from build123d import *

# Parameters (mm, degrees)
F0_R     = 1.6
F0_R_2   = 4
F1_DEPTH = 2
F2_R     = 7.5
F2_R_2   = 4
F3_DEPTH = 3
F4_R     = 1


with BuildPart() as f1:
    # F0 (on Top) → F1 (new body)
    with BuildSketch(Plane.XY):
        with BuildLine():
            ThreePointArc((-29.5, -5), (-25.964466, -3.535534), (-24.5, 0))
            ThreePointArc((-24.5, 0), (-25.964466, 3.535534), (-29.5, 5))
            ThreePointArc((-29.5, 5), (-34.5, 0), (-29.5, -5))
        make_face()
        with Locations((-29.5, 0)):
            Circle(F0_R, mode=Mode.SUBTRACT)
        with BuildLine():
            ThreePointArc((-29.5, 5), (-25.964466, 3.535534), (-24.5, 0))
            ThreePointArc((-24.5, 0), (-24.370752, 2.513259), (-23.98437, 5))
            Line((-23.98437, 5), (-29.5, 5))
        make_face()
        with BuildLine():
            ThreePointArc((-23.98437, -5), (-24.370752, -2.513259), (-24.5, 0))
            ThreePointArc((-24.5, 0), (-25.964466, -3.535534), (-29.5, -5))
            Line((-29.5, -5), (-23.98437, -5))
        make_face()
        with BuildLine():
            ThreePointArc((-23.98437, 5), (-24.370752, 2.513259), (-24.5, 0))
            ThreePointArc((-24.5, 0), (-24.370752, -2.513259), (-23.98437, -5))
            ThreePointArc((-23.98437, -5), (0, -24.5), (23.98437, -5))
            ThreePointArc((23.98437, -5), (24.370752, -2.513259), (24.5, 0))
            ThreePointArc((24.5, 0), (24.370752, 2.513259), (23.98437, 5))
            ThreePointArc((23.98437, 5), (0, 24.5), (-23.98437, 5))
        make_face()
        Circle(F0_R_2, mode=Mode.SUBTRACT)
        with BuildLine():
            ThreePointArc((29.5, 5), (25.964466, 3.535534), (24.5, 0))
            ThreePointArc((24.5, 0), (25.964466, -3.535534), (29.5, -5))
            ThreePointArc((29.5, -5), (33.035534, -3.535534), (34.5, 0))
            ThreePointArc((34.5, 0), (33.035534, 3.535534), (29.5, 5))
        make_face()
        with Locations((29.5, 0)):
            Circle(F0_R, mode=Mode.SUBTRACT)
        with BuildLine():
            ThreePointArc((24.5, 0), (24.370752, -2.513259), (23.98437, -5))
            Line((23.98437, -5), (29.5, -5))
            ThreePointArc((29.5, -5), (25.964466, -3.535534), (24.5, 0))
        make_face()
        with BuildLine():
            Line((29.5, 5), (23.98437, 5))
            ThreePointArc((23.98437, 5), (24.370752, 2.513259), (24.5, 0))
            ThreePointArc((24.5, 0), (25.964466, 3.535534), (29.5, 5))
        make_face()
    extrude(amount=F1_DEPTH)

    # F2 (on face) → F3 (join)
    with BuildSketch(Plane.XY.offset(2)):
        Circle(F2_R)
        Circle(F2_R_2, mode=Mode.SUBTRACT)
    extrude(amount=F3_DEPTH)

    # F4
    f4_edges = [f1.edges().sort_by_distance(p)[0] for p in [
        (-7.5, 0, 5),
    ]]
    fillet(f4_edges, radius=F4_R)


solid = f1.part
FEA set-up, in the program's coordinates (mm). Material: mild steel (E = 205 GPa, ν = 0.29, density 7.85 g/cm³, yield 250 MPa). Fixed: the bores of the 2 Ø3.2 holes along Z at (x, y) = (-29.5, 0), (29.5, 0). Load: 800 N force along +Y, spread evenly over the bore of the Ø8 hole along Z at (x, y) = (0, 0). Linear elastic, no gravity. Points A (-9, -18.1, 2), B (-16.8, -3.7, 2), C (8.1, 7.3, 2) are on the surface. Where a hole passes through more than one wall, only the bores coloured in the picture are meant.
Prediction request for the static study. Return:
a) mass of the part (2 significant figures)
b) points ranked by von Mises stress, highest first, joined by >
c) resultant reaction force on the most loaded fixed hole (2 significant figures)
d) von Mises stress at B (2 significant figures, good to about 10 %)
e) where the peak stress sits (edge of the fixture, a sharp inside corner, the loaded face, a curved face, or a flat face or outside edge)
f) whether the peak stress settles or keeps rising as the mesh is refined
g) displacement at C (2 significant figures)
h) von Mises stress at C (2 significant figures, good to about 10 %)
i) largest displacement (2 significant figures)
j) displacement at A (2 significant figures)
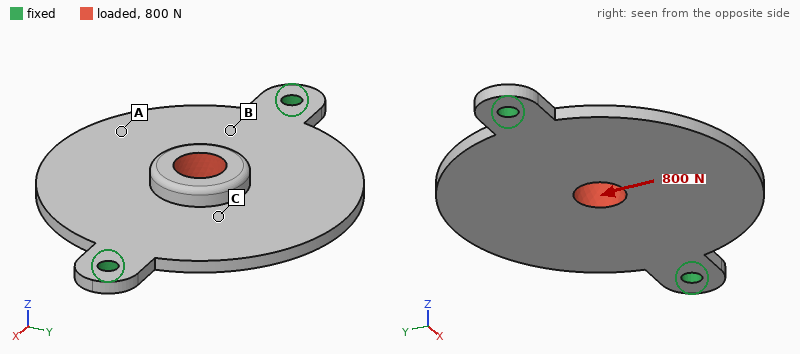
34 g
B > C > A
400 N
36 MPa
edge of the fixture
keeps rising
25 µm
21 MPa
81 µm
58 µm
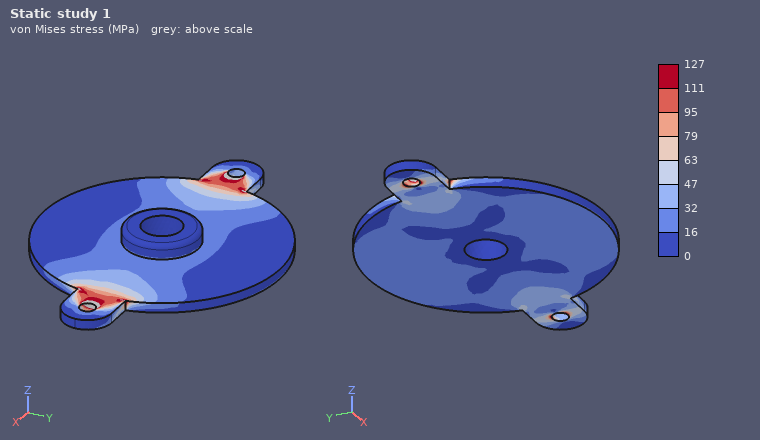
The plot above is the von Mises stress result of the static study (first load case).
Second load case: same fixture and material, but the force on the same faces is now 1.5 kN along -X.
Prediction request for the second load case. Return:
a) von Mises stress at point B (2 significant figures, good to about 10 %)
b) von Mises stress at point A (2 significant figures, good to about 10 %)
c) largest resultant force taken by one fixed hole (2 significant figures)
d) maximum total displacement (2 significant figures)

39 MPa
9.4 MPa
750 N
10 µm
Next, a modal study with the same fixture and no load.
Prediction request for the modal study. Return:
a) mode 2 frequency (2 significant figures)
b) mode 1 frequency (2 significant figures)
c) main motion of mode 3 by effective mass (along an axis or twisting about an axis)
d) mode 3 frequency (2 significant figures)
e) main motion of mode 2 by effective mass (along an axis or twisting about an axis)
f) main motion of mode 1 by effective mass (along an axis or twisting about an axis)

2100 Hz
1500 Hz
twisting about Y
5700 Hz
along Z
twisting about X
